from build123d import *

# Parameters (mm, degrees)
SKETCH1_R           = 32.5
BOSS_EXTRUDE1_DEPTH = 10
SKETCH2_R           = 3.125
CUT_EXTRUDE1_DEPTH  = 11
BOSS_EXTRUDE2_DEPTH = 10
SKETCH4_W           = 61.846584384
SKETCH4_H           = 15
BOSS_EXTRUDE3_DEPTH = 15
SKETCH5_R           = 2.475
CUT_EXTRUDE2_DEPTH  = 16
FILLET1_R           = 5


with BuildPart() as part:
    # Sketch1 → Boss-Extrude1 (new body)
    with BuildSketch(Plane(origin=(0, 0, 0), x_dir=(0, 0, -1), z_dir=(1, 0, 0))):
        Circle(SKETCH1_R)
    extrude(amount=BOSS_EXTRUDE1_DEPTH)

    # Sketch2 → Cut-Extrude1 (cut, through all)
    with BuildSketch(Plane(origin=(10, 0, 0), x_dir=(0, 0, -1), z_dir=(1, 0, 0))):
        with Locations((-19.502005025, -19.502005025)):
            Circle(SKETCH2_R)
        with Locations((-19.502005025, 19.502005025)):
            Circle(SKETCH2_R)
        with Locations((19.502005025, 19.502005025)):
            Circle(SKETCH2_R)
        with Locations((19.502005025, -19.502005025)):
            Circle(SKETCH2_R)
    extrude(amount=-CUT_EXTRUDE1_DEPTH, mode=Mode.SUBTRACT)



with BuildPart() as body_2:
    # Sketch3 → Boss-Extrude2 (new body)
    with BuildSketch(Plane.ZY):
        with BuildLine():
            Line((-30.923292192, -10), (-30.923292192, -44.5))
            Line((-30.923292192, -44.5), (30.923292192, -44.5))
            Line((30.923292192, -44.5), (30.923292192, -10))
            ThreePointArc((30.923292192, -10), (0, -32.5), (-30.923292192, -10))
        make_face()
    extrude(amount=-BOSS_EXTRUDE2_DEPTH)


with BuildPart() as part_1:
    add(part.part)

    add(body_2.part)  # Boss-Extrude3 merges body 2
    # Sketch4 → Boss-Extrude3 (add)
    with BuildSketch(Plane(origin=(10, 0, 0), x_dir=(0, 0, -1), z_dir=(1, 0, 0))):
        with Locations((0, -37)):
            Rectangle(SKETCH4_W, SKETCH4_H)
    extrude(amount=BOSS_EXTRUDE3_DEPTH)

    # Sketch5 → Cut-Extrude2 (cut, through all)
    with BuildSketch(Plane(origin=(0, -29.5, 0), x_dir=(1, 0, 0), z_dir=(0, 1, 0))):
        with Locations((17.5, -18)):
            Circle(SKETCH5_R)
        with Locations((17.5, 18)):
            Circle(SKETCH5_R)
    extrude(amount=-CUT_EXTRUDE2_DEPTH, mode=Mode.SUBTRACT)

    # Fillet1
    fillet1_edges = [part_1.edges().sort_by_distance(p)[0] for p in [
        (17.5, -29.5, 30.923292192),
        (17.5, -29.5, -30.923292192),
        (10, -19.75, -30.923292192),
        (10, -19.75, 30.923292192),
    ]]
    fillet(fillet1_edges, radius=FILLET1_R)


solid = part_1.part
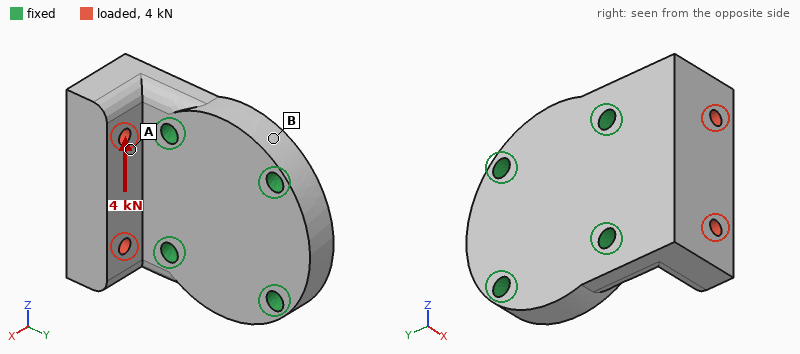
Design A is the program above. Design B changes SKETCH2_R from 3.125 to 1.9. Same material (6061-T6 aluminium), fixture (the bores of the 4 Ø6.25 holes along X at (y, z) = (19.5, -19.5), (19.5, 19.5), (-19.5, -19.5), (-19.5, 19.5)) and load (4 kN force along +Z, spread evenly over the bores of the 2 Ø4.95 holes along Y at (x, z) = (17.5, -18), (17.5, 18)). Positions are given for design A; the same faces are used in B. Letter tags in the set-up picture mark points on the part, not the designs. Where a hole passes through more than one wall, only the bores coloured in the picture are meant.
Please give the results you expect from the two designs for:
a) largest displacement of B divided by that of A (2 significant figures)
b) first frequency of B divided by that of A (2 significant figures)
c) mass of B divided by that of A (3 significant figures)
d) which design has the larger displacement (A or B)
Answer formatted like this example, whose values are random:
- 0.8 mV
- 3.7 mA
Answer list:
- 1.2
- 0.89
- 1.01
- B
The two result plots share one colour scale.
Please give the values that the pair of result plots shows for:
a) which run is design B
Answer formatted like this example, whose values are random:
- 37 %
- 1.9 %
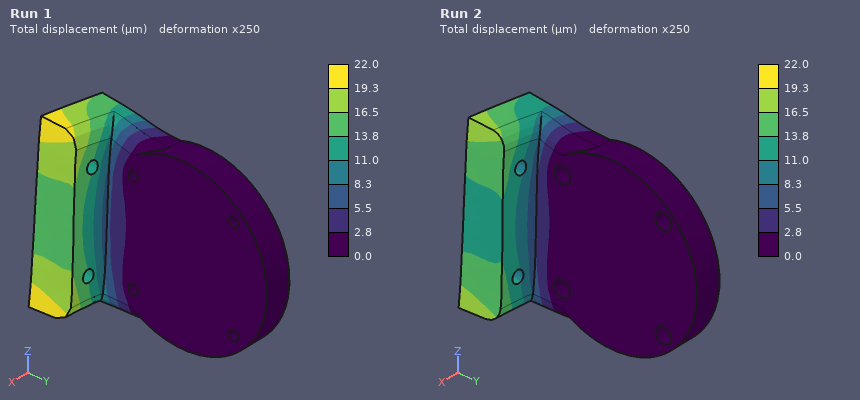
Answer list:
- Run 1
